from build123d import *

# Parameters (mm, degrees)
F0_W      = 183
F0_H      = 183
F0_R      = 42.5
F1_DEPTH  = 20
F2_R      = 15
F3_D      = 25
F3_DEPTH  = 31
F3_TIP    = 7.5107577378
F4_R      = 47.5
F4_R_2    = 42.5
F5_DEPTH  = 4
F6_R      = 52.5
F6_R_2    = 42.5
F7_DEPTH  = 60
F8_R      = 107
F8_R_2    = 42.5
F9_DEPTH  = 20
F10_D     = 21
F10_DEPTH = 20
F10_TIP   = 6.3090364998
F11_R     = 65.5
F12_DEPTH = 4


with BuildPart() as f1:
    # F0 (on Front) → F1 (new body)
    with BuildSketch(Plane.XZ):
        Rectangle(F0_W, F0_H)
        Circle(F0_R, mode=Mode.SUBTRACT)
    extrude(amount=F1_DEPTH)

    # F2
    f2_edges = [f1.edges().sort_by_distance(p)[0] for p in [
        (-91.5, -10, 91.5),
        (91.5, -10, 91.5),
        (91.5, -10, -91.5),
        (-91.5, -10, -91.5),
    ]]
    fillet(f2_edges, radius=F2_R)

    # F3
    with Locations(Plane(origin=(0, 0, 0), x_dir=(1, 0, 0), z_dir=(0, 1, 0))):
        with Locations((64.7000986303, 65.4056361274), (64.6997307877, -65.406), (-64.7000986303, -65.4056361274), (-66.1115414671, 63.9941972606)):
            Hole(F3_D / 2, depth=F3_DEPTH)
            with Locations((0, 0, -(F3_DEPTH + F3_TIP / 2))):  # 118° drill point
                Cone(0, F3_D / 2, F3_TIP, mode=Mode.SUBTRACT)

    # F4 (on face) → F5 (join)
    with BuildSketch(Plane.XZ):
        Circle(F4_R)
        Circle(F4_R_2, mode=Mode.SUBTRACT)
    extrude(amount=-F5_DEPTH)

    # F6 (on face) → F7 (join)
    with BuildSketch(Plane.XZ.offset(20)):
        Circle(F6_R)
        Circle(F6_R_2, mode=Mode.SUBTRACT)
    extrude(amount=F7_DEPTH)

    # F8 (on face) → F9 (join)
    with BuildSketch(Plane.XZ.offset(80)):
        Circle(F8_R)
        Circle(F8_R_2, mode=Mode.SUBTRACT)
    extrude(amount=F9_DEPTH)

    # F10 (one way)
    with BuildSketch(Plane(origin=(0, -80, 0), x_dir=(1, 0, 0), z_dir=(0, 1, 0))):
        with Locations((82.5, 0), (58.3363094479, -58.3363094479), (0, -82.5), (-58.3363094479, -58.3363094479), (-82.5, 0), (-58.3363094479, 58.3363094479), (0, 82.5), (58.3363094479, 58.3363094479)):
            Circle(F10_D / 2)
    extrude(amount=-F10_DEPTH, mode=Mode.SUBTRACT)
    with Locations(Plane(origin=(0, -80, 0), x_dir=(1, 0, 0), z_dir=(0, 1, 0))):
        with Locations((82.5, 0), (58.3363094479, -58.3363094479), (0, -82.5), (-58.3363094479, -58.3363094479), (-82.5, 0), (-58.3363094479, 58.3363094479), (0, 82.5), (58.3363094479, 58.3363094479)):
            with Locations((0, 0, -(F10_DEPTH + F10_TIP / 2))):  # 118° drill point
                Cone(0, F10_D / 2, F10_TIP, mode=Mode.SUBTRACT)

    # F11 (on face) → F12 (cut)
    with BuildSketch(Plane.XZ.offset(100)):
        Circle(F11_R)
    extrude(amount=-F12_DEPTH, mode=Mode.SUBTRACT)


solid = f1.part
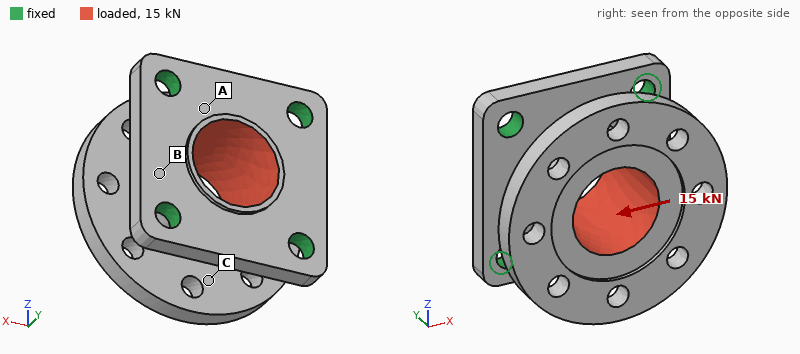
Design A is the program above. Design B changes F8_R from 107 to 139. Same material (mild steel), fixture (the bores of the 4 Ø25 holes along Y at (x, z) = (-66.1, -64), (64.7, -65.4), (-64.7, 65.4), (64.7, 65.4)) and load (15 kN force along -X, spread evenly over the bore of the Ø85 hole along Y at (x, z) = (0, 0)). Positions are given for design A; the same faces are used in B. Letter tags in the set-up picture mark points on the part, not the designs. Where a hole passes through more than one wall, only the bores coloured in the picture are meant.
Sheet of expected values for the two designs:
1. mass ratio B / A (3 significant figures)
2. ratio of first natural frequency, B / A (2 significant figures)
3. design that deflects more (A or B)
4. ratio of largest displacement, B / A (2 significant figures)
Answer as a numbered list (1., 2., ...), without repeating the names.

1. 1.41
2. 0.57
3. B
4. 1.1
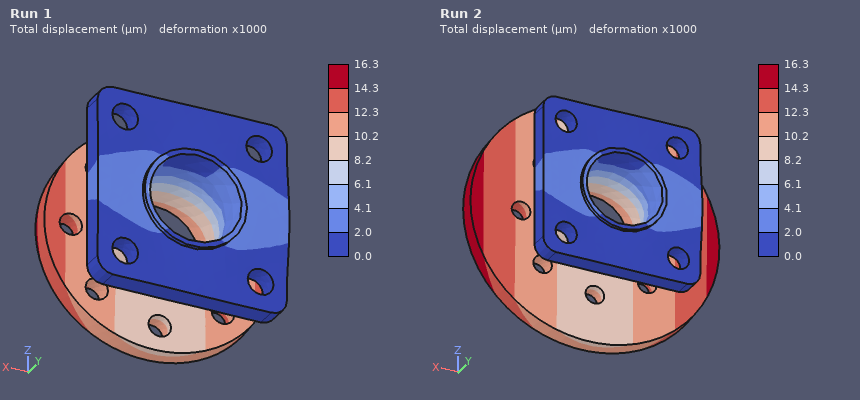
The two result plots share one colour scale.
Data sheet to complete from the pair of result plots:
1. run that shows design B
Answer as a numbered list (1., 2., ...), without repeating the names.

1. Run 2
